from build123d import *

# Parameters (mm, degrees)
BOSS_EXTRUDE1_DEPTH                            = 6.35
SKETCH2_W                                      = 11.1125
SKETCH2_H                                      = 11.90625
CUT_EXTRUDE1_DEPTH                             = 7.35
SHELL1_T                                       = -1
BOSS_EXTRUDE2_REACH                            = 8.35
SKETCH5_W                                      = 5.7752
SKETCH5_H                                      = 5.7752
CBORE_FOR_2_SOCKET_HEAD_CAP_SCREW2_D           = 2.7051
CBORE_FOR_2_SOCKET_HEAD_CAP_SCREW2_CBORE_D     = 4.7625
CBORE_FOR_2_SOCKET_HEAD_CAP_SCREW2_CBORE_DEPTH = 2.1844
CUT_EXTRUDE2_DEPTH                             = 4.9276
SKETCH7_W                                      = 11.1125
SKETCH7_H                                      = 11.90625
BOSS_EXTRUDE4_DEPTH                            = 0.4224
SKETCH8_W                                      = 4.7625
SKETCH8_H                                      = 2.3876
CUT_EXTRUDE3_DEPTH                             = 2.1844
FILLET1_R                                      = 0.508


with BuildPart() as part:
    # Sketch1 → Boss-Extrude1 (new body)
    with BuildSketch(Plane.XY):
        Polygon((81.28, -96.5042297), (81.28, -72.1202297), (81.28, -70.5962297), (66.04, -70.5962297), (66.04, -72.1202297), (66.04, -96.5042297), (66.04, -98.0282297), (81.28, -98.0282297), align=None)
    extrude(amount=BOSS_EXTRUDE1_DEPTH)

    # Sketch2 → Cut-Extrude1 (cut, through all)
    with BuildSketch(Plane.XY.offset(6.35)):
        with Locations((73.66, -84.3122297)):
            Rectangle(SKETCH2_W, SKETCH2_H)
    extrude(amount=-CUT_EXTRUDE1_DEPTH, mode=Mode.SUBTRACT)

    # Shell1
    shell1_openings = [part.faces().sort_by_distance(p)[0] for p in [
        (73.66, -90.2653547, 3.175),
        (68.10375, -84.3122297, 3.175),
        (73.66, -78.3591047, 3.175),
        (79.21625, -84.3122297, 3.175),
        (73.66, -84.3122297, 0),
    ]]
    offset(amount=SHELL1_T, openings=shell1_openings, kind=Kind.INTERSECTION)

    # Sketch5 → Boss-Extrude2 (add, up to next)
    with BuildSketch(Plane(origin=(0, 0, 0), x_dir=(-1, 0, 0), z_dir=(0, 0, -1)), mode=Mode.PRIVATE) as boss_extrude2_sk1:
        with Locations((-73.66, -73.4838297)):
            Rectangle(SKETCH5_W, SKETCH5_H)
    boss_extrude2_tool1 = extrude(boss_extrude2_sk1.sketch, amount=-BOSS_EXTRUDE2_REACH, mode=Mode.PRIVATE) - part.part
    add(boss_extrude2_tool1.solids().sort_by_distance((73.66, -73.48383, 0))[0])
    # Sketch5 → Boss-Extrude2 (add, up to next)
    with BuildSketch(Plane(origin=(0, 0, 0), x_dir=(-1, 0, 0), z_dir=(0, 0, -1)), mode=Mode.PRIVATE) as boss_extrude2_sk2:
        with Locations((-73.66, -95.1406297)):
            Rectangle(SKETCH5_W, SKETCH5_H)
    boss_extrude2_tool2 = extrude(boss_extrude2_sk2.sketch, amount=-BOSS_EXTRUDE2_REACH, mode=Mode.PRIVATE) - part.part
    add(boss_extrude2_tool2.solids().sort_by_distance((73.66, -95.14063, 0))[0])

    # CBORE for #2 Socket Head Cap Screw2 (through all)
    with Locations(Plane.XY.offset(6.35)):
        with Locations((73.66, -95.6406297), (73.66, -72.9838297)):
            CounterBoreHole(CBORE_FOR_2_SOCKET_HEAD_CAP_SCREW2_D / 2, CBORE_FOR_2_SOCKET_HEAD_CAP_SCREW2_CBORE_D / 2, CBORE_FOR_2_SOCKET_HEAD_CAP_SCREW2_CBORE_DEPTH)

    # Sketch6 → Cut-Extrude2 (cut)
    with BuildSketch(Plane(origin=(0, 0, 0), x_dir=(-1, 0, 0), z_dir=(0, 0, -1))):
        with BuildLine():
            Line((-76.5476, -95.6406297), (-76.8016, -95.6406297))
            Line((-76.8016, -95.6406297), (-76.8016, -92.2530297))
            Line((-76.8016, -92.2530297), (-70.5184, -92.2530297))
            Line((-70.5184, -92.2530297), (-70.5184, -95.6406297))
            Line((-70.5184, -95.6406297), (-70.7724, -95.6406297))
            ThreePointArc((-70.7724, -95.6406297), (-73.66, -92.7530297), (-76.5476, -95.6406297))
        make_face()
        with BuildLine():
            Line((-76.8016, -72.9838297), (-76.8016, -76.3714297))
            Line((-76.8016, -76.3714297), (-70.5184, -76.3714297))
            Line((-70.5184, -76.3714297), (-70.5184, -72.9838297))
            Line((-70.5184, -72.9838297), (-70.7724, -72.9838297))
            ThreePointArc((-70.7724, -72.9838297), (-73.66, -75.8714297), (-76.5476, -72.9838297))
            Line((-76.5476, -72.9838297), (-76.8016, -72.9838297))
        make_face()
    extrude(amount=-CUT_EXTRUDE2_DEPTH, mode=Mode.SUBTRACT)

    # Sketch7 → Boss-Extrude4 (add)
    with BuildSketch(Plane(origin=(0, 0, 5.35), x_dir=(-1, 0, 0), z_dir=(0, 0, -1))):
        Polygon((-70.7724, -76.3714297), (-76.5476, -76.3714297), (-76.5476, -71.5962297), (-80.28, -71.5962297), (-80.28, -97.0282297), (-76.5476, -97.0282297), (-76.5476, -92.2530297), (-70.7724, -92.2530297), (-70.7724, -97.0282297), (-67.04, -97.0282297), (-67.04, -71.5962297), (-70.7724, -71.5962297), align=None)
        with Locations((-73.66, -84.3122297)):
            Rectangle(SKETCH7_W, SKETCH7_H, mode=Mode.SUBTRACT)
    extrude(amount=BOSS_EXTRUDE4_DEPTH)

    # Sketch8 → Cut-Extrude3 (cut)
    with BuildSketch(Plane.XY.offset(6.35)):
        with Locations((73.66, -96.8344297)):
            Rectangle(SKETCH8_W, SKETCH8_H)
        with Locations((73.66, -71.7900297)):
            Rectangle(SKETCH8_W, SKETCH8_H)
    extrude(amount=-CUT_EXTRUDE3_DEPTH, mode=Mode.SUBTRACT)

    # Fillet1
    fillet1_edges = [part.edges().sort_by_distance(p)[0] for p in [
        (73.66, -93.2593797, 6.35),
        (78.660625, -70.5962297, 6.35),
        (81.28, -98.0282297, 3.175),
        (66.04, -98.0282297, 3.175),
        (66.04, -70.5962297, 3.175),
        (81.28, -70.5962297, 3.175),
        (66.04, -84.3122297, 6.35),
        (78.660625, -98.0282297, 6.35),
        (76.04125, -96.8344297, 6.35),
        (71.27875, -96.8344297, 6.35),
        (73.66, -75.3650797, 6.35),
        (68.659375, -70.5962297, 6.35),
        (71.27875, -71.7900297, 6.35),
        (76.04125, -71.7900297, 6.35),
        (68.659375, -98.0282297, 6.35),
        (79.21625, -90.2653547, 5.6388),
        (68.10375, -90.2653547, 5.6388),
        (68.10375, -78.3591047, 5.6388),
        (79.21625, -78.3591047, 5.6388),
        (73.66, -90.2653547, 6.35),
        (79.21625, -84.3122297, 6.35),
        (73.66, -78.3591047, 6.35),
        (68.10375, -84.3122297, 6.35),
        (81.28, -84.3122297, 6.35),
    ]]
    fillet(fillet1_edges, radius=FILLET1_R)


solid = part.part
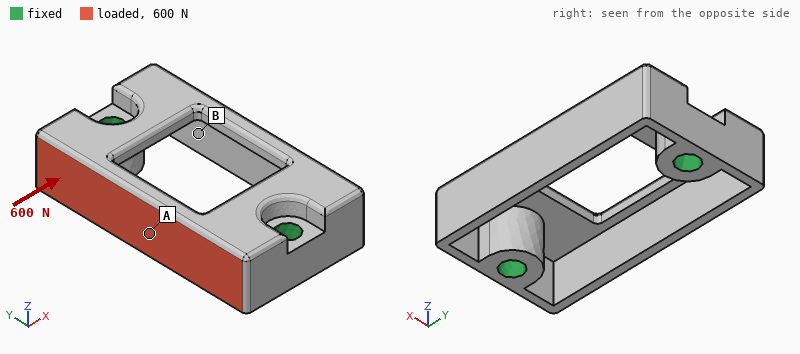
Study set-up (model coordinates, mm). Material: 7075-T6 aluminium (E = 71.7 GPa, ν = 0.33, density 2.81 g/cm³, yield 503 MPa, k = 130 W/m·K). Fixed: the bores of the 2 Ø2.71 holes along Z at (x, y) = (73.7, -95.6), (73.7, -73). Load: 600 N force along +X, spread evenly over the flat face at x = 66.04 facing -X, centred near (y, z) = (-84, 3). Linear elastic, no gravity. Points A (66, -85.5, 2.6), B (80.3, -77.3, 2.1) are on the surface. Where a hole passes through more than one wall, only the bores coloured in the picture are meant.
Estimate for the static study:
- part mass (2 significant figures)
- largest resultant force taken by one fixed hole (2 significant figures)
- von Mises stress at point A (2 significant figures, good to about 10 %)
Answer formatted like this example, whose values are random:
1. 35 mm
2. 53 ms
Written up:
1. 2.4 g
2. 320 N
3. 130 MPa
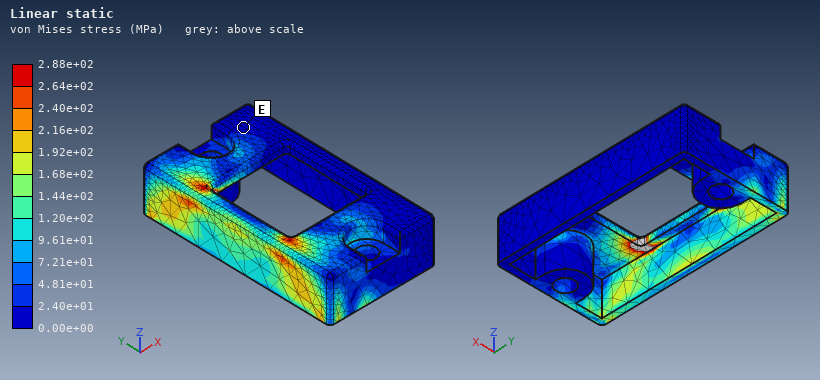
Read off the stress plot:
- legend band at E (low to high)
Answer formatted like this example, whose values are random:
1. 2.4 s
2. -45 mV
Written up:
1. 0.00e+00 to 2.40e+01 MPa
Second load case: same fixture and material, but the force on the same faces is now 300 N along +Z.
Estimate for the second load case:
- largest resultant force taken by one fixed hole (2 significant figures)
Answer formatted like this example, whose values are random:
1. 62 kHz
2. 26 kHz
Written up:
1. 160 N
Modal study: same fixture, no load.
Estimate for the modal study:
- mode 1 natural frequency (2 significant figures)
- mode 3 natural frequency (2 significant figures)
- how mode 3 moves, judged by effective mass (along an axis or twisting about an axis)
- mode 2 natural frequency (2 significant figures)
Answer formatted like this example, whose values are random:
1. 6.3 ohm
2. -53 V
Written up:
1. 15 kHz
2. 19 kHz
3. along X
4. 15 kHz
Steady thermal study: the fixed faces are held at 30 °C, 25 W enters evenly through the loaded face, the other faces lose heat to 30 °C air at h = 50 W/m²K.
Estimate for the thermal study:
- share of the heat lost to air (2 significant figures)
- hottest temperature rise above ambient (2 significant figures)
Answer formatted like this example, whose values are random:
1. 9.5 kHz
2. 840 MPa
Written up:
1. 5.9 %
2. 88 K
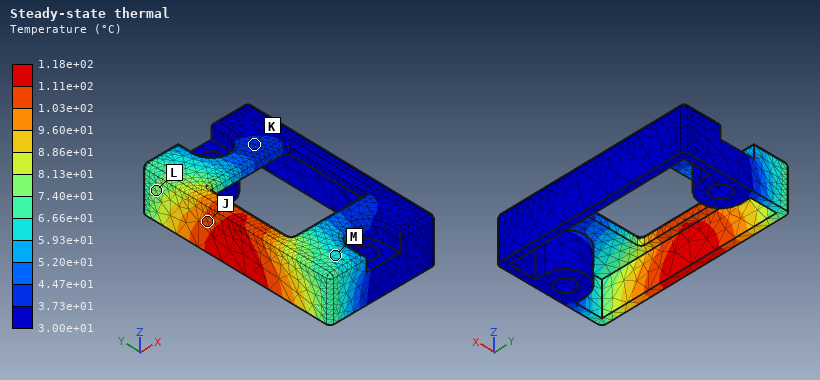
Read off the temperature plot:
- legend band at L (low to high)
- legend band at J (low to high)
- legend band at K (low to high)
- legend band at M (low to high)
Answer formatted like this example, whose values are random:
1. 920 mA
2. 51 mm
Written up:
1. 7.40e+01 to 8.13e+01 °C
2. 1.03e+02 to 1.11e+02 °C
3. 3.73e+01 to 4.47e+01 °C
4. 5.93e+01 to 6.66e+01 °C
